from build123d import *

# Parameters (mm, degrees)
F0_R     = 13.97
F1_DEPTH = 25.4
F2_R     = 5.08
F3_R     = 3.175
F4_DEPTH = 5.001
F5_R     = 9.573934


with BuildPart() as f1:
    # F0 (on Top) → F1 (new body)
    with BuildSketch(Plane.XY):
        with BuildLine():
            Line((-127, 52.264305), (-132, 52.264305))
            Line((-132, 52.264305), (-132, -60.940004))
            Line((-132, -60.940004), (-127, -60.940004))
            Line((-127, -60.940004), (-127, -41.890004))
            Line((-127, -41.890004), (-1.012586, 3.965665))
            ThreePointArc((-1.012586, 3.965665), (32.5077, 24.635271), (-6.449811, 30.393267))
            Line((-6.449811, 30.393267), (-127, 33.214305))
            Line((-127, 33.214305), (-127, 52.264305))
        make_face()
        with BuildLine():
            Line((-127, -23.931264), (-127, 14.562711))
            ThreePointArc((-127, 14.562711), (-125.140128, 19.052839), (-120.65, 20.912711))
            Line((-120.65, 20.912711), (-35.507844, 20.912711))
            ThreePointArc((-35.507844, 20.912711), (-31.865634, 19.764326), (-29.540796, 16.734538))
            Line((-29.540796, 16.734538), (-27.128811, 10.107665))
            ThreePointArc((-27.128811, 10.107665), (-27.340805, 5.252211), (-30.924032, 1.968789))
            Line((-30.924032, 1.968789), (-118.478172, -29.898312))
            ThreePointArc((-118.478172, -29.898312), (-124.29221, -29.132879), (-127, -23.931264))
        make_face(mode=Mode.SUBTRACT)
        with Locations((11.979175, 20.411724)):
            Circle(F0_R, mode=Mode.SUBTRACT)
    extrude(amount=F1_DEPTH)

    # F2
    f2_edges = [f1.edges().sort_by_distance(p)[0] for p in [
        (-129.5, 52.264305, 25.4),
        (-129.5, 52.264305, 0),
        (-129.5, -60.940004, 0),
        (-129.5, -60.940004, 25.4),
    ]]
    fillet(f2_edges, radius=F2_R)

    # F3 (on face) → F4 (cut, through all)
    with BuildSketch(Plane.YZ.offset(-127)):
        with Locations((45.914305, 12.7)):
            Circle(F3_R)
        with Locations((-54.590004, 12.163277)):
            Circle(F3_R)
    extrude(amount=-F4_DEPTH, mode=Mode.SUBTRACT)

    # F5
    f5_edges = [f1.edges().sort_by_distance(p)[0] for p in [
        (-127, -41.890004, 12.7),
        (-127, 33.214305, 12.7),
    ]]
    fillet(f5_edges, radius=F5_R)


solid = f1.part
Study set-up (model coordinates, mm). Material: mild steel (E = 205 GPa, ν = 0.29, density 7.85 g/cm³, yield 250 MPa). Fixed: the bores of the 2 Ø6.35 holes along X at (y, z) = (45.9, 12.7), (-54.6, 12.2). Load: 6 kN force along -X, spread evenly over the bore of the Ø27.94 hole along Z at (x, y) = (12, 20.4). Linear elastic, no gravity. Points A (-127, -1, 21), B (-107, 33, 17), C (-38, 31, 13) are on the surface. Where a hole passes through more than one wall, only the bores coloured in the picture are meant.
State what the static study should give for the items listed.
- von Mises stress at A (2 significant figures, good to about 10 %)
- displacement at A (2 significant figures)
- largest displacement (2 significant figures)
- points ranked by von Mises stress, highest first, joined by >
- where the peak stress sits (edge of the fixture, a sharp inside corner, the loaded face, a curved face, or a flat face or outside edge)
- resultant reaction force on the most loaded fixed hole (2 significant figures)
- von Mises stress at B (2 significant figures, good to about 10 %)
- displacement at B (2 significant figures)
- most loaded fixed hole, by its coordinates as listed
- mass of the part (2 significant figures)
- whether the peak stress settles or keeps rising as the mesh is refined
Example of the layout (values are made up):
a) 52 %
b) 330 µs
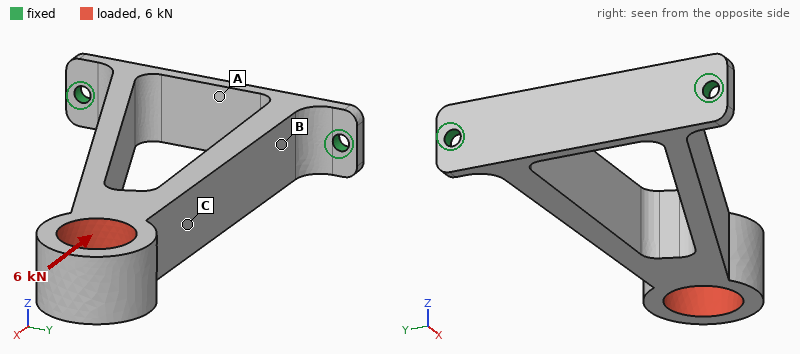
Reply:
a) 33 MPa
b) 51 µm
c) 84 µm
d) B > A > C
e) edge of the fixture
f) 4.8 kN
g) 71 MPa
h) 41 µm
i) (45.9, 12.7)
j) 810 g
k) keeps rising
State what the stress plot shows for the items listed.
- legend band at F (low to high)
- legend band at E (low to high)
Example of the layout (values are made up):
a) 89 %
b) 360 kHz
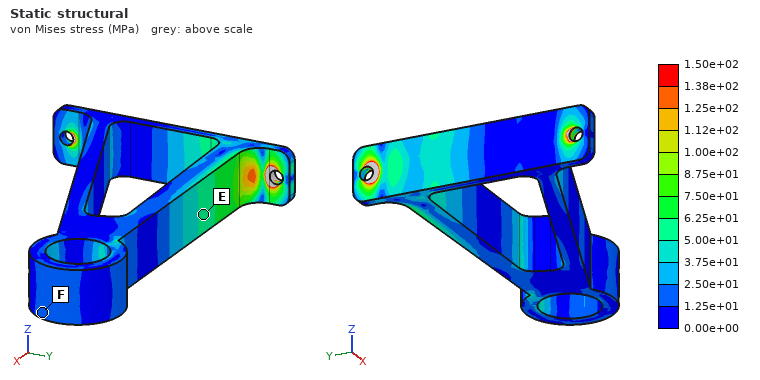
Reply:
a) 1.25e+01 to 2.50e+01 MPa
b) 5.00e+01 to 6.25e+01 MPa
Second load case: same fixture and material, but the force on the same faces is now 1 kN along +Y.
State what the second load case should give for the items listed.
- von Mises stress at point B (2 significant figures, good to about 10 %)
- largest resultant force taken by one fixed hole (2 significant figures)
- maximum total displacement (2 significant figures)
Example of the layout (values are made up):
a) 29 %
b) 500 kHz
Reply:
a) 24 MPa
b) 1.7 kN
c) 74 µm
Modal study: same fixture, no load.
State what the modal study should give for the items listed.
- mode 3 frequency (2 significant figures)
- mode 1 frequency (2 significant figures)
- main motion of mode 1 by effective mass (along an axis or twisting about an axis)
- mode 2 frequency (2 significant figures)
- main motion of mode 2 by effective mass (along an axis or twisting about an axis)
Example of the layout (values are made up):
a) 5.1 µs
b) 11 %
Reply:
a) 1700 Hz
b) 270 Hz
c) along Z
d) 1100 Hz
e) along Y
